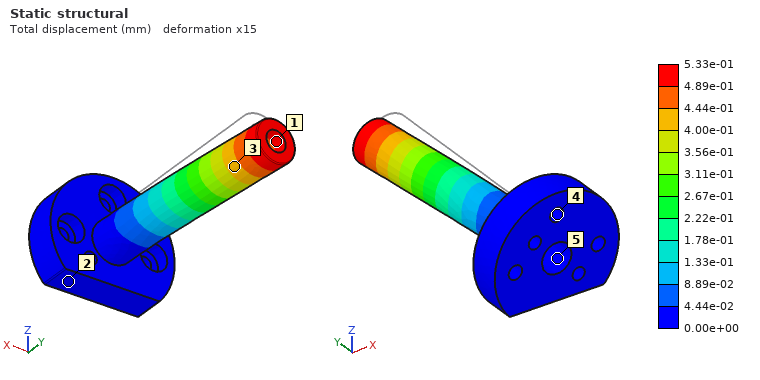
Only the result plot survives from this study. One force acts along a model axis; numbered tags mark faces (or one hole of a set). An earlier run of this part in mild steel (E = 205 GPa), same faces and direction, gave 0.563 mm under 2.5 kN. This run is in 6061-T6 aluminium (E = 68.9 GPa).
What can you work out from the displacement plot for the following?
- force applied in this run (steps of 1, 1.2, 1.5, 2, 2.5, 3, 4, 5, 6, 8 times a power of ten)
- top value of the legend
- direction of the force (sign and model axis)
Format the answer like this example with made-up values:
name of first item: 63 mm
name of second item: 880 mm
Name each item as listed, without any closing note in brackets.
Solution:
force applied in this run: 800 N
top value of the legend: 5.33e-01 mm
direction of the force: -X
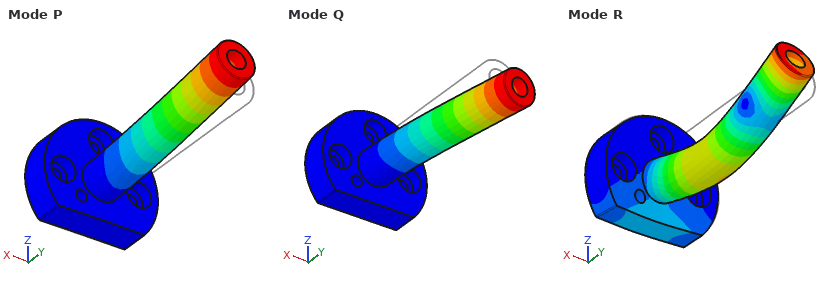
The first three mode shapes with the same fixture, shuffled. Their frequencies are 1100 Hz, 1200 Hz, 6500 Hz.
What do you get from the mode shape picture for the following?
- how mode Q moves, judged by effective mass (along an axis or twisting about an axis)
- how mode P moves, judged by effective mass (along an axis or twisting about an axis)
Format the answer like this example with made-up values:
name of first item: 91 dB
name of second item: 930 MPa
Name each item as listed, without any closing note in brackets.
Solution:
how mode Q moves, judged by effective mass: along X
how mode P moves, judged by effective mass: along Z
